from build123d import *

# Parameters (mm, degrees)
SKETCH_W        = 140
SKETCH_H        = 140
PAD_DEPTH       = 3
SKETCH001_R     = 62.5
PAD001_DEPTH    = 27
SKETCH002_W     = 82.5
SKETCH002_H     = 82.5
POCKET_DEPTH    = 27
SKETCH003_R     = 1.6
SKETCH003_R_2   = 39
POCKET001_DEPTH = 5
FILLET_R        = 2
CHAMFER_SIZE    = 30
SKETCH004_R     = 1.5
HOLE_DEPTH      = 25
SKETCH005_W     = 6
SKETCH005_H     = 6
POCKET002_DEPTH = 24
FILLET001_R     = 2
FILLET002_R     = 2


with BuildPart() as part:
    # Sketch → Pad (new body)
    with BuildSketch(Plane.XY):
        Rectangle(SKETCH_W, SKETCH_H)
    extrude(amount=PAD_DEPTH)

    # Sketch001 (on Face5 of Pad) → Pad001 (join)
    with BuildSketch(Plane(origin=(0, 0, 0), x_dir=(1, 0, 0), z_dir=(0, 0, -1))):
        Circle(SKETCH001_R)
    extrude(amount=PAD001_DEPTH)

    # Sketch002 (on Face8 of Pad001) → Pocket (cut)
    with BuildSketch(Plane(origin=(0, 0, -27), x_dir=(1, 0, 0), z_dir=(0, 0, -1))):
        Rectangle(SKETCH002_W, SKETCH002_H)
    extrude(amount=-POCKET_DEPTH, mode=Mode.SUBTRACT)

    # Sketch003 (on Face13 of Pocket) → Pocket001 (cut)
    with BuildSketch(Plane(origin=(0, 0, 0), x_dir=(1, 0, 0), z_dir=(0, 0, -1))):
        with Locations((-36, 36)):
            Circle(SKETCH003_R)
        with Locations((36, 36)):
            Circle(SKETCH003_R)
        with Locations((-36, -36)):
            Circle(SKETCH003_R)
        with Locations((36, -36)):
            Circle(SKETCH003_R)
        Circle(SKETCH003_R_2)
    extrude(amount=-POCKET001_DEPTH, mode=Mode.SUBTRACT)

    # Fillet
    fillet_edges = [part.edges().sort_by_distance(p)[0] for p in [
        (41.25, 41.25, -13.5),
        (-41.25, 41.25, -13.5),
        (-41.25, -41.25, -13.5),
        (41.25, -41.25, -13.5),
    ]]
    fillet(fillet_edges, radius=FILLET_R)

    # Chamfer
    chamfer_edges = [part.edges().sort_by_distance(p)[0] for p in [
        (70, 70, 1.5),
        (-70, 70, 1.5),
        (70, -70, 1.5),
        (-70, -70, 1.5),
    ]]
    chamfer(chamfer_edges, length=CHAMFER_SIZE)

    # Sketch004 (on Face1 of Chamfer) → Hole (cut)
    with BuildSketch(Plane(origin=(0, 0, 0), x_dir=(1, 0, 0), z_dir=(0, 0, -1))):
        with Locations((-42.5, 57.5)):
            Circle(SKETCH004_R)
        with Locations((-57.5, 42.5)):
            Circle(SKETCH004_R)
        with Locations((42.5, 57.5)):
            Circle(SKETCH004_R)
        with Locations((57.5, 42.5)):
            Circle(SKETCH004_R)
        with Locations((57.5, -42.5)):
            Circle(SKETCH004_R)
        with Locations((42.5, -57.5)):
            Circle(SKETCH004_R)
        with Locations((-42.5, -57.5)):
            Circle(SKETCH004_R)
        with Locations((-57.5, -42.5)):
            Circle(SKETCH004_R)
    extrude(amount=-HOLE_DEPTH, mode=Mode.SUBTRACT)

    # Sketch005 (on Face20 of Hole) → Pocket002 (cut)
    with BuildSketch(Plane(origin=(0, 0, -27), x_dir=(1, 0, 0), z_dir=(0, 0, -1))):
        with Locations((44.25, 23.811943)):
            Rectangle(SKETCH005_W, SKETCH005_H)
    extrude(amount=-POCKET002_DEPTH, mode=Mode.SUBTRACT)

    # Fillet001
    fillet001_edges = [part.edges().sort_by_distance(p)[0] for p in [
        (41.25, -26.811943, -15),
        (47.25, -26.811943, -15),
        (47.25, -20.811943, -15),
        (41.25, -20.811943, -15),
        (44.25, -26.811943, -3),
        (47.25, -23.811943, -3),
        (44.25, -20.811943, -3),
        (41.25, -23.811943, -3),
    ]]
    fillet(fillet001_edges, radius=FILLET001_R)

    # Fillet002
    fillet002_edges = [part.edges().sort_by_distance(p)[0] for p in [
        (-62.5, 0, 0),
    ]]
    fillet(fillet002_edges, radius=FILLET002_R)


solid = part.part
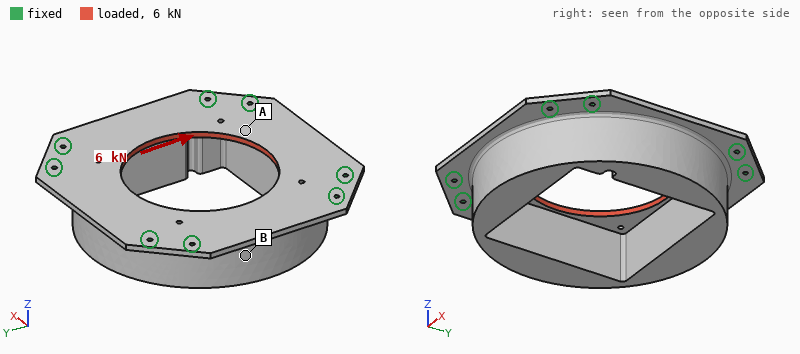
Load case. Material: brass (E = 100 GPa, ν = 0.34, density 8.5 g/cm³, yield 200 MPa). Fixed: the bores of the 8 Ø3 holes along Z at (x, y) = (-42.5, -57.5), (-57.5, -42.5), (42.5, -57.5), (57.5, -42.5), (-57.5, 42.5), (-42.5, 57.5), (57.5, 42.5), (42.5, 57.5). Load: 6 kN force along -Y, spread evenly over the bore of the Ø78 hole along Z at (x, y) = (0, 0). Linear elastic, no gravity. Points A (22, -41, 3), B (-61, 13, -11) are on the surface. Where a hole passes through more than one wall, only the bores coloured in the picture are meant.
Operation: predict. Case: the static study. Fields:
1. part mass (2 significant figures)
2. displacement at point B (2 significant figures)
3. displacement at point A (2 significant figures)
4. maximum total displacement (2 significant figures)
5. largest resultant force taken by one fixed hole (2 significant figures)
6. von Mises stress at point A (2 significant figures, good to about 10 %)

1.6 kg
2.7 µm
6.1 µm
8.6 µm
910 N
8.4 MPa
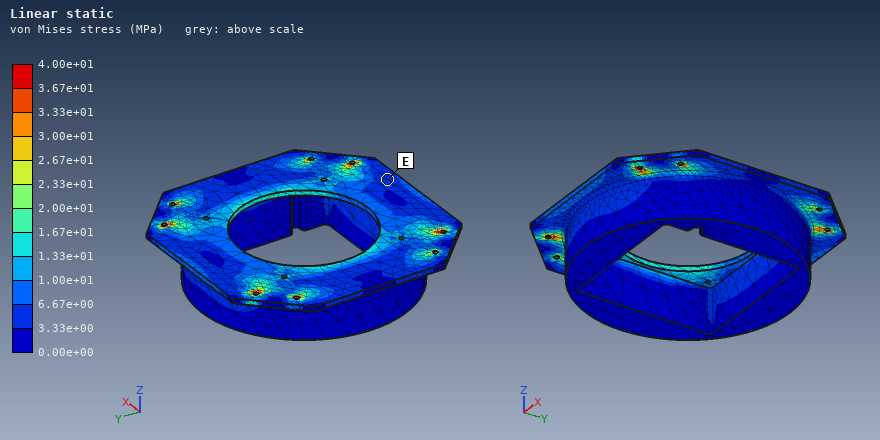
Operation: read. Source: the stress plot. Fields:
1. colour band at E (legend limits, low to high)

3.33e+00 to 6.67e+00 MPa
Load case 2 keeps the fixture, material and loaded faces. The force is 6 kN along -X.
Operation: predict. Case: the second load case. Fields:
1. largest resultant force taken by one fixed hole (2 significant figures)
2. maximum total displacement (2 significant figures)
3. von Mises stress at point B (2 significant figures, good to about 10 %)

920 N
8.8 µm
3.9 MPa
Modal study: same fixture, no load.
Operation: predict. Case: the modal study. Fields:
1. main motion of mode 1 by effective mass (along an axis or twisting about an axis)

along Z
